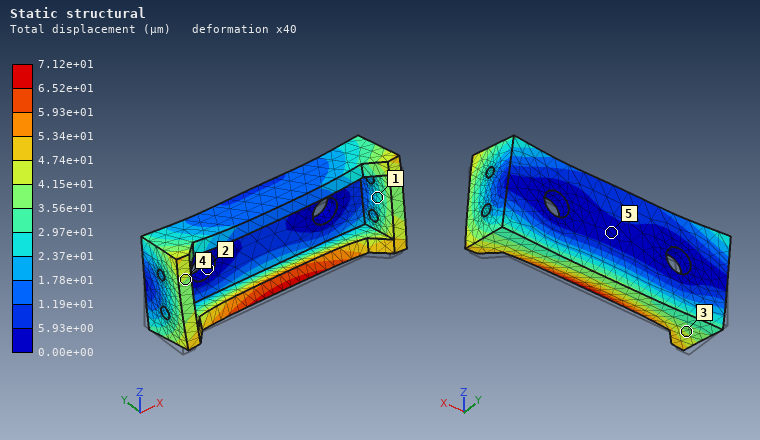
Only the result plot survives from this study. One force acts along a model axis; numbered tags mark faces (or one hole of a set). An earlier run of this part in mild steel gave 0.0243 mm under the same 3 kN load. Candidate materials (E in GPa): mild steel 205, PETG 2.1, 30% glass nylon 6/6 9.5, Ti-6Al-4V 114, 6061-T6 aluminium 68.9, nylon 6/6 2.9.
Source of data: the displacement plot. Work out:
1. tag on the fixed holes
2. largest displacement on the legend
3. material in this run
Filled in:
2
7.12e+01 µm
6061-T6 aluminium
